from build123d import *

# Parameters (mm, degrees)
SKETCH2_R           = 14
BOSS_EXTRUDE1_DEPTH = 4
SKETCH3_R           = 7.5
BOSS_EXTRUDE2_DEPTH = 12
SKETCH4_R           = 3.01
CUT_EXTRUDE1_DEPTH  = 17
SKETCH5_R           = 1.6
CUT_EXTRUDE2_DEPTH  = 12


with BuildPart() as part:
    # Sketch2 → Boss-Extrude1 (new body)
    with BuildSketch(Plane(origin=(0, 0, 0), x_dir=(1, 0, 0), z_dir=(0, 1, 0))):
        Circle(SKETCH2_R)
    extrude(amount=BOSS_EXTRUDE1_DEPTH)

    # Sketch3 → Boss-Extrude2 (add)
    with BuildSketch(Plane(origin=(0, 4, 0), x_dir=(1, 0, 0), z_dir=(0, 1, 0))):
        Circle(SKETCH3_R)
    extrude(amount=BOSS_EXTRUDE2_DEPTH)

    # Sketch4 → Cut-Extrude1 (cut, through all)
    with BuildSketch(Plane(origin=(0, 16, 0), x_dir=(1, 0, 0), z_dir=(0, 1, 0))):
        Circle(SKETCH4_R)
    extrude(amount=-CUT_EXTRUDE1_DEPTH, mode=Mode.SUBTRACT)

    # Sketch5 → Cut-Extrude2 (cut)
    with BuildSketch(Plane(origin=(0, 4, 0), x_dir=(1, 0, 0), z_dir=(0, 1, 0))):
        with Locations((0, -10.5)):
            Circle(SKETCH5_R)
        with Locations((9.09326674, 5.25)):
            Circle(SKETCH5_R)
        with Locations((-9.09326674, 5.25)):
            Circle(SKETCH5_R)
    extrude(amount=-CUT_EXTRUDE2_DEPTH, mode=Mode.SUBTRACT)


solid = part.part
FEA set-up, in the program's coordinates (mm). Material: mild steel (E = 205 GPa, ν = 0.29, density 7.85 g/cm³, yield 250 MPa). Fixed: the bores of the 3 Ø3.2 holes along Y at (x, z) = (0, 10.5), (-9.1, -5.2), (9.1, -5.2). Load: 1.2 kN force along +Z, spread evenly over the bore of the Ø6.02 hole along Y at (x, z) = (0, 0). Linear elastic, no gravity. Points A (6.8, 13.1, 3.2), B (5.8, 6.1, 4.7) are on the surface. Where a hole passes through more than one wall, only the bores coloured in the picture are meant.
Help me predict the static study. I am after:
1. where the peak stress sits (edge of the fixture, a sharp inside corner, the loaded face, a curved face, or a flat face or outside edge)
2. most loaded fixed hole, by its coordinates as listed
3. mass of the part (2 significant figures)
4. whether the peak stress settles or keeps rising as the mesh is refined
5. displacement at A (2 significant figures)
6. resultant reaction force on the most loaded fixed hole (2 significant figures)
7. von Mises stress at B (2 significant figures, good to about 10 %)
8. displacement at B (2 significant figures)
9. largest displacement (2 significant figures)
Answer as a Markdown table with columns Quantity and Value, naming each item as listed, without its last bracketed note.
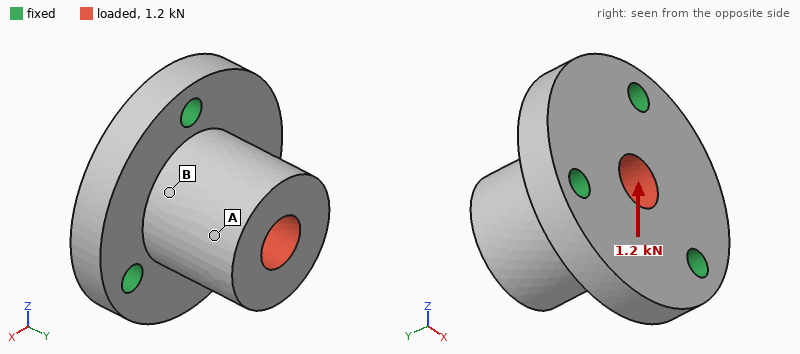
| Quantity | Value |
|---|---|
| where the peak stress sits | edge of the fixture |
| most loaded fixed hole, by its coordinates as listed | (0, 10.5) |
| mass of the part | 32 g |
| whether the peak stress settles or keeps rising as the mesh is refined | keeps rising |
| displacement at A | 2.4 µm |
| resultant reaction force on the most loaded fixed hole | 660 N |
| von Mises stress at B | 11 MPa |
| displacement at B | 1.1 µm |
| largest displacement | 3.2 µm |
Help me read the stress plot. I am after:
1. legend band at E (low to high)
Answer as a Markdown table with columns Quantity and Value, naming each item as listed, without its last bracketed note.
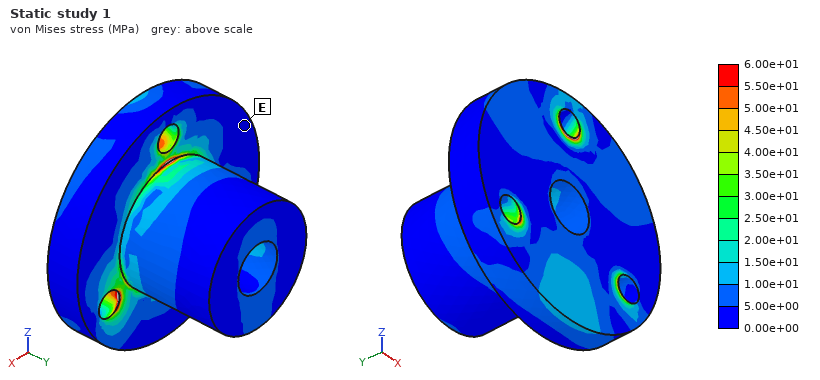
| Quantity | Value |
|---|---|
| legend band at E | 0.00e+00 to 5.00e+00 MPa |
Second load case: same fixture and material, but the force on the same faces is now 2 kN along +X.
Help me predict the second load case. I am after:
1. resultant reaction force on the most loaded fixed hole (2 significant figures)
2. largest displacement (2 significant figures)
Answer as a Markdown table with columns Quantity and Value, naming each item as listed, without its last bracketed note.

| Quantity | Value |
|---|---|
| resultant reaction force on the most loaded fixed hole | 990 N |
| largest displacement | 5.3 µm |
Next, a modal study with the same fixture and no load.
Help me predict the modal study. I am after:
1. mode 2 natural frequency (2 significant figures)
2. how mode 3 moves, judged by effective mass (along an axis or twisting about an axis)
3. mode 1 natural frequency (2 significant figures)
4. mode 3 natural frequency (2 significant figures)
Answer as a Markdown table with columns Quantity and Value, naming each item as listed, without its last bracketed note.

| Quantity | Value |
|---|---|
| mode 2 natural frequency | 25 kHz |
| how mode 3 moves, judged by effective mass | along Y |
| mode 1 natural frequency | 25 kHz |
| mode 3 natural frequency | 36 kHz |
